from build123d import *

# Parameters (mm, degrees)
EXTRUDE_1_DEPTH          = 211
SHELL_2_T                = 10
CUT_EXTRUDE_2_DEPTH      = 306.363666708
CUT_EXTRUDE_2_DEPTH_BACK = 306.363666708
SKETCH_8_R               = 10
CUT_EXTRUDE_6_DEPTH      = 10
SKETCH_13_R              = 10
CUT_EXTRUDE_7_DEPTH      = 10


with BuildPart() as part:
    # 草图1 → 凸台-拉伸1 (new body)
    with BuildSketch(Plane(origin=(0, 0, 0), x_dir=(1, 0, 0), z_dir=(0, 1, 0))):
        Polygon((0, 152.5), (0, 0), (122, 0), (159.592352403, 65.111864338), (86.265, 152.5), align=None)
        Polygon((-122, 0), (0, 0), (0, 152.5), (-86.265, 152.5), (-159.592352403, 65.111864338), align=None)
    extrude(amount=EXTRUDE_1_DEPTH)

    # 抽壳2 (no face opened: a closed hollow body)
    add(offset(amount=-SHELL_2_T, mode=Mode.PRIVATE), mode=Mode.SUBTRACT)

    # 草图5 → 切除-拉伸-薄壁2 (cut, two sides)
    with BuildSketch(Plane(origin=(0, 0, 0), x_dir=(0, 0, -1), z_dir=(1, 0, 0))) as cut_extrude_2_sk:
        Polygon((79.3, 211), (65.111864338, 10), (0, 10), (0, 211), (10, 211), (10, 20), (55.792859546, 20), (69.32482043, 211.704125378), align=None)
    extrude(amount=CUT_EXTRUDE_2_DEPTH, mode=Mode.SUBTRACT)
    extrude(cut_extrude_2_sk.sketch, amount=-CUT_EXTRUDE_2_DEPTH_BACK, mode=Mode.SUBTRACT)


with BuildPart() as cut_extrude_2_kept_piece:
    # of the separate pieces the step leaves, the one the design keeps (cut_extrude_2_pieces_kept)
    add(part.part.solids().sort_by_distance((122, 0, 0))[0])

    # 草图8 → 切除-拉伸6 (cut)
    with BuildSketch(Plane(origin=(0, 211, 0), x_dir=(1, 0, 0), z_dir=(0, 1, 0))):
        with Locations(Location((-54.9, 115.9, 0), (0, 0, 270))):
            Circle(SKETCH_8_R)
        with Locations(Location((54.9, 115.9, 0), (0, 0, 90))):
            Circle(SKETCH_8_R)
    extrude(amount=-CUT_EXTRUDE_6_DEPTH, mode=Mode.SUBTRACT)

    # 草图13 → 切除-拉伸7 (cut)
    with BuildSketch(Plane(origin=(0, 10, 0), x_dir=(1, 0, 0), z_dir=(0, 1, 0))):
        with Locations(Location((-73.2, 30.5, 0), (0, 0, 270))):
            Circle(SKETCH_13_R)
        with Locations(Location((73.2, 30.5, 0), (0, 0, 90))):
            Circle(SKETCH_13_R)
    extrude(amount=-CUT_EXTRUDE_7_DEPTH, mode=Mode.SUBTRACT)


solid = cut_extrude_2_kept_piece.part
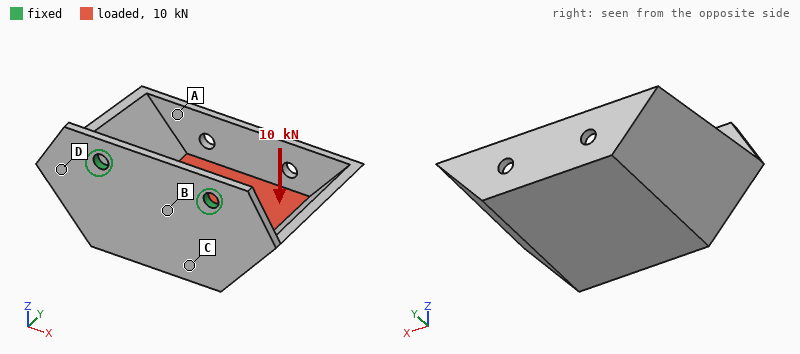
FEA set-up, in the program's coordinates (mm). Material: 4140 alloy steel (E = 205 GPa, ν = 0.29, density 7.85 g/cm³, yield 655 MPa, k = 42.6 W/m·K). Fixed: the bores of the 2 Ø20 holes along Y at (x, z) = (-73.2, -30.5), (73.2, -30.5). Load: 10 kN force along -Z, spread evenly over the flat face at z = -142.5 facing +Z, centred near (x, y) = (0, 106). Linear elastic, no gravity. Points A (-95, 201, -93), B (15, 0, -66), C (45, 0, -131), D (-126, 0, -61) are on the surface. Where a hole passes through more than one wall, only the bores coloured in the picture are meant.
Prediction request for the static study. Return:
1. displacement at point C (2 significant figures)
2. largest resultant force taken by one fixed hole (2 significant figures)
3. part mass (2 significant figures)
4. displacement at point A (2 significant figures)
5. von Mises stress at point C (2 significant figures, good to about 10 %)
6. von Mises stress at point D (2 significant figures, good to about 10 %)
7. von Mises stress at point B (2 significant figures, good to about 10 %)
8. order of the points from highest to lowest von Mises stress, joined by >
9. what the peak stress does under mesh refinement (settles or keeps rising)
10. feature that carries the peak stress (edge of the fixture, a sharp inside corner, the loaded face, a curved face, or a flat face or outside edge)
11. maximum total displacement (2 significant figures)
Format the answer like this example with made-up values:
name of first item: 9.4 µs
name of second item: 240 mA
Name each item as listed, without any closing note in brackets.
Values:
displacement at point C: 0.94 mm
largest resultant force taken by one fixed hole: 5.0 kN
part mass: 9.9 kg
displacement at point A: 3.2 mm
von Mises stress at point C: 66 MPa
von Mises stress at point D: 210 MPa
von Mises stress at point B: 130 MPa
order of the points from highest to lowest von Mises stress, joined by >: D > B > C > A
what the peak stress does under mesh refinement: keeps rising
feature that carries the peak stress: edge of the fixture
maximum total displacement: 3.6 mm
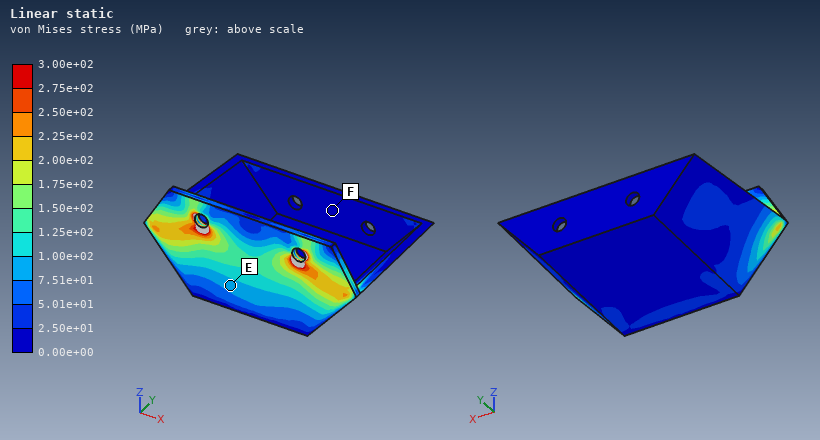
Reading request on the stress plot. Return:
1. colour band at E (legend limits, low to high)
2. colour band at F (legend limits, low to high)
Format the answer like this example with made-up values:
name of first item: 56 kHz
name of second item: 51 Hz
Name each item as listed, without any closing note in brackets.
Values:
colour band at E: 7.51e+01 to 1.00e+02 MPa
colour band at F: 0.00e+00 to 2.50e+01 MPa
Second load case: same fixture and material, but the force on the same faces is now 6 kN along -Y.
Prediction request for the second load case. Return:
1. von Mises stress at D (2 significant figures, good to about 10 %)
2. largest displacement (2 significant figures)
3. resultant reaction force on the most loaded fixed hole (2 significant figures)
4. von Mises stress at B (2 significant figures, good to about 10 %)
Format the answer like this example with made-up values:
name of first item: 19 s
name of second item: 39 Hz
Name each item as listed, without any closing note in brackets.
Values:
von Mises stress at D: 87 MPa
largest displacement: 1.5 mm
resultant reaction force on the most loaded fixed hole: 3.0 kN
von Mises stress at B: 69 MPa
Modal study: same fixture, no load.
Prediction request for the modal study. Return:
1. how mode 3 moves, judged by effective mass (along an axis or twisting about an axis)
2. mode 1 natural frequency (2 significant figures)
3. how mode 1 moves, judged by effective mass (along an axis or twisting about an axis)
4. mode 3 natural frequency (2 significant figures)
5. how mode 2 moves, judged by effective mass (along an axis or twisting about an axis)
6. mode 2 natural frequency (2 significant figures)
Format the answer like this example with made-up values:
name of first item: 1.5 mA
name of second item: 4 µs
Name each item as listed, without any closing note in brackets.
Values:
how mode 3 moves, judged by effective mass: along Y
mode 1 natural frequency: 100 Hz
how mode 1 moves, judged by effective mass: along Z
mode 3 natural frequency: 440 Hz
how mode 2 moves, judged by effective mass: along X
mode 2 natural frequency: 180 Hz
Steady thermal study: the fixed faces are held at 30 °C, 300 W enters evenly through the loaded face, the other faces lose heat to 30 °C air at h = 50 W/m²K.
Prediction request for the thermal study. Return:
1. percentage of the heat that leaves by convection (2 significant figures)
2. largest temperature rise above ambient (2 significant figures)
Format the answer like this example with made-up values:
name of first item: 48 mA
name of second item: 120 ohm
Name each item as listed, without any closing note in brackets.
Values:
percentage of the heat that leaves by convection: 95 %
largest temperature rise above ambient: 78 K
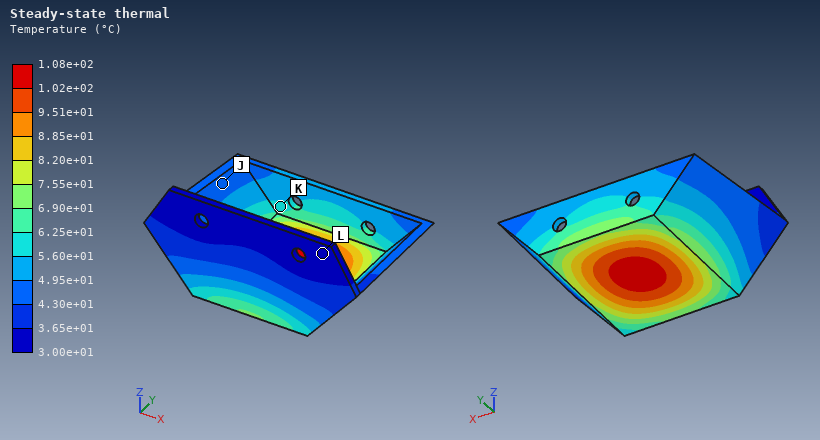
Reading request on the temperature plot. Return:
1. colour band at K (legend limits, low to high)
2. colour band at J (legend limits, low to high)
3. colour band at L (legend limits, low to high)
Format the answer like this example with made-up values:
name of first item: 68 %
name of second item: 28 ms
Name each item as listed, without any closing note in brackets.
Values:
colour band at K: 5.60e+01 to 6.25e+01 °C
colour band at J: 4.30e+01 to 4.95e+01 °C
colour band at L: 3.00e+01 to 3.65e+01 °C
